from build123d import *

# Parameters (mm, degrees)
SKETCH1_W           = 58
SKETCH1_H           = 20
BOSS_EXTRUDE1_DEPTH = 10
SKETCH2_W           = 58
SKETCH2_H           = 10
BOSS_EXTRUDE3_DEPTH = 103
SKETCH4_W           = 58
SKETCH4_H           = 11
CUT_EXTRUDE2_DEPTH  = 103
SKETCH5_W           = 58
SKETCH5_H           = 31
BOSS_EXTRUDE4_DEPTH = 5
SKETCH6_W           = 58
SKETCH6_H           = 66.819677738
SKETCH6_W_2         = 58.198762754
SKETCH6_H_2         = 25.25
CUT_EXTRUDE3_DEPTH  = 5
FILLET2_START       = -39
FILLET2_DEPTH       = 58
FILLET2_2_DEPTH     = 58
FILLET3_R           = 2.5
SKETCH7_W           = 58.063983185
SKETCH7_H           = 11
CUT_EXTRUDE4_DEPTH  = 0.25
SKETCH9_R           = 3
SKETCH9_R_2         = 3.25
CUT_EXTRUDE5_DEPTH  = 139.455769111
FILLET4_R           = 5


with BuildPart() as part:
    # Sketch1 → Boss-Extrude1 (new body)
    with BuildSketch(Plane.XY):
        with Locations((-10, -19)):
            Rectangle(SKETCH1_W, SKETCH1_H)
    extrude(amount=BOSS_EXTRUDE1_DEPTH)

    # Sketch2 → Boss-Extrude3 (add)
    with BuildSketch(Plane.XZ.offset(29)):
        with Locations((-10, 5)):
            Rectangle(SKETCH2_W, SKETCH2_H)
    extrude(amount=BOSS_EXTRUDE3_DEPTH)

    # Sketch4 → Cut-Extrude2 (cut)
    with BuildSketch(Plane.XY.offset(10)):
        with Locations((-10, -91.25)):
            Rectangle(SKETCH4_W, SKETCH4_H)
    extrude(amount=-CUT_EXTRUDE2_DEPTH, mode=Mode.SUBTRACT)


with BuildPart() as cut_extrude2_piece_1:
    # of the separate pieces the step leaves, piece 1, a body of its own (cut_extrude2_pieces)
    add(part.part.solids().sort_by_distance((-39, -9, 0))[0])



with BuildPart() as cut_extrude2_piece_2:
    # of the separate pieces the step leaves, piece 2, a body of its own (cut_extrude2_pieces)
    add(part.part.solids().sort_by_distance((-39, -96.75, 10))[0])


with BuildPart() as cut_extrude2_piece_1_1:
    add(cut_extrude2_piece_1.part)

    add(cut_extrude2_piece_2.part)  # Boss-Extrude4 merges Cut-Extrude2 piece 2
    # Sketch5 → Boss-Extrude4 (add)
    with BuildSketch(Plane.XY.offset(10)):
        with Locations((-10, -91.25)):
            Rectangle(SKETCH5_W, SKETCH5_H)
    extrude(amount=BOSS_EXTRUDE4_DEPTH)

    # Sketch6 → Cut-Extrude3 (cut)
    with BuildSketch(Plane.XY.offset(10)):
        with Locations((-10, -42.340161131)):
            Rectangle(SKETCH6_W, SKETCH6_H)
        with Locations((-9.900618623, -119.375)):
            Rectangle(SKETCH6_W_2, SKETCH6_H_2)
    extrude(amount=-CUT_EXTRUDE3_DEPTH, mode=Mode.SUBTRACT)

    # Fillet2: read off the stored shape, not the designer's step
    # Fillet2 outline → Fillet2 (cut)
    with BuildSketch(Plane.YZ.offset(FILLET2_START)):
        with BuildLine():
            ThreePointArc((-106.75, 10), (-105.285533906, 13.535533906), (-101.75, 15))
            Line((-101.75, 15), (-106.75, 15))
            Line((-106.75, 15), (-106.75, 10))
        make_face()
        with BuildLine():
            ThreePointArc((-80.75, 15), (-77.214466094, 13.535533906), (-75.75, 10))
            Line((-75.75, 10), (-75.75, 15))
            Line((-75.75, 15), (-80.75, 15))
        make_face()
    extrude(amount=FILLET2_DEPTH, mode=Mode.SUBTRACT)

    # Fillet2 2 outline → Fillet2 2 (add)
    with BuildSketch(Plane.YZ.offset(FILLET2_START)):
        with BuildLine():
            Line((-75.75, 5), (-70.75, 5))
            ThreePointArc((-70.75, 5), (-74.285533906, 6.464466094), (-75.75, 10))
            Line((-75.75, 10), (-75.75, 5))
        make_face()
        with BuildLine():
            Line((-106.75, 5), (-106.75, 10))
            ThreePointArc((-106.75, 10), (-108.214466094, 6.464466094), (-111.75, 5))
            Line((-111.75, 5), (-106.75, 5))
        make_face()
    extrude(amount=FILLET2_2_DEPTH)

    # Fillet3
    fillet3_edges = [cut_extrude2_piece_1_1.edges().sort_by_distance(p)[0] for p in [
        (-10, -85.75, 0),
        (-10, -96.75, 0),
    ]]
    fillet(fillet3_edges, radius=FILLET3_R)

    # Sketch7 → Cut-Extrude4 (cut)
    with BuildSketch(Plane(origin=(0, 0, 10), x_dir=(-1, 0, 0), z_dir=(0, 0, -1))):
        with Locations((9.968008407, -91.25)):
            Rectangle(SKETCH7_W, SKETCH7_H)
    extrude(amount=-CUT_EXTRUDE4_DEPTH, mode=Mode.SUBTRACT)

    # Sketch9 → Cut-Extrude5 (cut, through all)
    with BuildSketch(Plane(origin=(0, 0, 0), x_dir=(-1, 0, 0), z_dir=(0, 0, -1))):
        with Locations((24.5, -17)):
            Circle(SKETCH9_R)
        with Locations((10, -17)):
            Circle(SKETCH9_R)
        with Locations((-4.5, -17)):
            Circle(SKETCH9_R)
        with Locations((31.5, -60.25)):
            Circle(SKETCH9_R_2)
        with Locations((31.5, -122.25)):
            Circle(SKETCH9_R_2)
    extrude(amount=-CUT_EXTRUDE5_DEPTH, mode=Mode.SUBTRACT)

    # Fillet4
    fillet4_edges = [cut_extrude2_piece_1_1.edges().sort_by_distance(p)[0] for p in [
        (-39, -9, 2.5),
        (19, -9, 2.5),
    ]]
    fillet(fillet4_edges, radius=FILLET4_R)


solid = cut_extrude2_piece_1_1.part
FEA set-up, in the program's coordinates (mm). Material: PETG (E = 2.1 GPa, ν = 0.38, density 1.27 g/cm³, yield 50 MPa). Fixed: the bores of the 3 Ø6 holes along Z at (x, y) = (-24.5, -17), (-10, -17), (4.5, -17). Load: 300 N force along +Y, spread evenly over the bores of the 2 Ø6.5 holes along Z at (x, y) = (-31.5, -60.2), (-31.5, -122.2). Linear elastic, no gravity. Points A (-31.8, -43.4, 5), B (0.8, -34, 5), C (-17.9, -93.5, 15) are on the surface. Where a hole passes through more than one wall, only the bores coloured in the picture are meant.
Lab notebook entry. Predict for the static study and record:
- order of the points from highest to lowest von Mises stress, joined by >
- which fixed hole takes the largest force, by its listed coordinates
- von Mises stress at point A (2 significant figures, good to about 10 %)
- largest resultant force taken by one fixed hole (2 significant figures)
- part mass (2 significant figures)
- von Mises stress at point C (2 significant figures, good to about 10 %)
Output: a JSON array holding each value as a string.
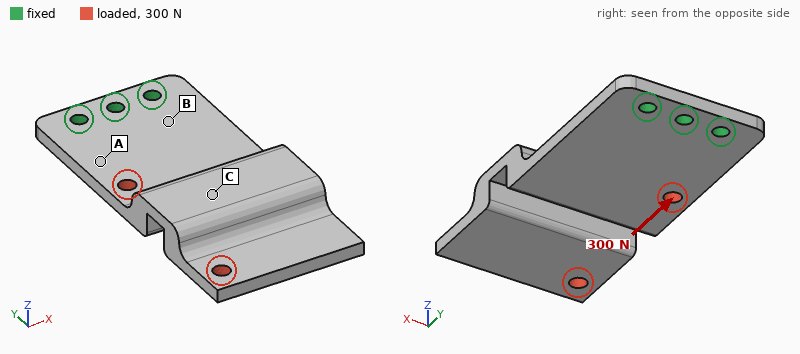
["C > A > B", "(-24.5, -17)", "2.8 MPa", "300 N", "59 g", "6.2 MPa"]
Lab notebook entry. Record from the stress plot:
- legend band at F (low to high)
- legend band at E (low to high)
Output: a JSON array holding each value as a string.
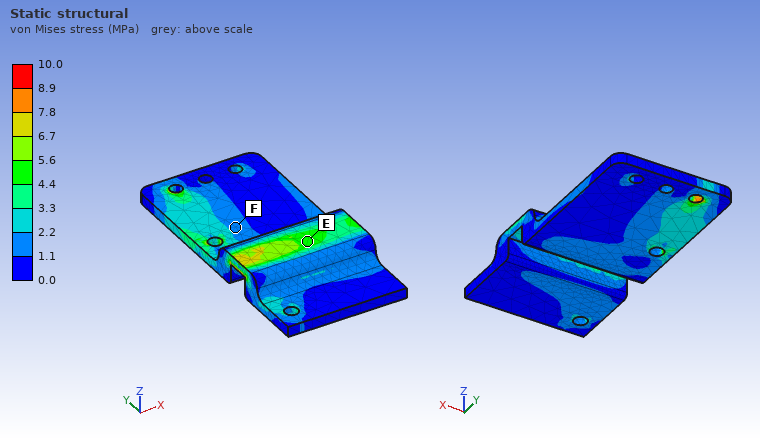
["1.1 to 2.2 MPa", "4.4 to 5.6 MPa"]
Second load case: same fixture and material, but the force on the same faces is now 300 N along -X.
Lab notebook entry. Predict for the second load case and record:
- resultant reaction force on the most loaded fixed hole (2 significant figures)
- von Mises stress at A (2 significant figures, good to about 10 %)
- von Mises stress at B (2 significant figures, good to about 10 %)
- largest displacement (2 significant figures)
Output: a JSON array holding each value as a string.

["660 N", "4.0 MPa", "4.6 MPa", "1.2 mm"]
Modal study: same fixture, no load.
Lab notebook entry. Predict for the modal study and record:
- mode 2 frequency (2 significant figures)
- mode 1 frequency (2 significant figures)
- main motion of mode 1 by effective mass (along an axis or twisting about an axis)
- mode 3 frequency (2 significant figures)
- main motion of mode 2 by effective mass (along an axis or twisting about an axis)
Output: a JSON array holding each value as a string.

["300 Hz", "71 Hz", "along Z", "480 Hz", "twisting about Y"]
